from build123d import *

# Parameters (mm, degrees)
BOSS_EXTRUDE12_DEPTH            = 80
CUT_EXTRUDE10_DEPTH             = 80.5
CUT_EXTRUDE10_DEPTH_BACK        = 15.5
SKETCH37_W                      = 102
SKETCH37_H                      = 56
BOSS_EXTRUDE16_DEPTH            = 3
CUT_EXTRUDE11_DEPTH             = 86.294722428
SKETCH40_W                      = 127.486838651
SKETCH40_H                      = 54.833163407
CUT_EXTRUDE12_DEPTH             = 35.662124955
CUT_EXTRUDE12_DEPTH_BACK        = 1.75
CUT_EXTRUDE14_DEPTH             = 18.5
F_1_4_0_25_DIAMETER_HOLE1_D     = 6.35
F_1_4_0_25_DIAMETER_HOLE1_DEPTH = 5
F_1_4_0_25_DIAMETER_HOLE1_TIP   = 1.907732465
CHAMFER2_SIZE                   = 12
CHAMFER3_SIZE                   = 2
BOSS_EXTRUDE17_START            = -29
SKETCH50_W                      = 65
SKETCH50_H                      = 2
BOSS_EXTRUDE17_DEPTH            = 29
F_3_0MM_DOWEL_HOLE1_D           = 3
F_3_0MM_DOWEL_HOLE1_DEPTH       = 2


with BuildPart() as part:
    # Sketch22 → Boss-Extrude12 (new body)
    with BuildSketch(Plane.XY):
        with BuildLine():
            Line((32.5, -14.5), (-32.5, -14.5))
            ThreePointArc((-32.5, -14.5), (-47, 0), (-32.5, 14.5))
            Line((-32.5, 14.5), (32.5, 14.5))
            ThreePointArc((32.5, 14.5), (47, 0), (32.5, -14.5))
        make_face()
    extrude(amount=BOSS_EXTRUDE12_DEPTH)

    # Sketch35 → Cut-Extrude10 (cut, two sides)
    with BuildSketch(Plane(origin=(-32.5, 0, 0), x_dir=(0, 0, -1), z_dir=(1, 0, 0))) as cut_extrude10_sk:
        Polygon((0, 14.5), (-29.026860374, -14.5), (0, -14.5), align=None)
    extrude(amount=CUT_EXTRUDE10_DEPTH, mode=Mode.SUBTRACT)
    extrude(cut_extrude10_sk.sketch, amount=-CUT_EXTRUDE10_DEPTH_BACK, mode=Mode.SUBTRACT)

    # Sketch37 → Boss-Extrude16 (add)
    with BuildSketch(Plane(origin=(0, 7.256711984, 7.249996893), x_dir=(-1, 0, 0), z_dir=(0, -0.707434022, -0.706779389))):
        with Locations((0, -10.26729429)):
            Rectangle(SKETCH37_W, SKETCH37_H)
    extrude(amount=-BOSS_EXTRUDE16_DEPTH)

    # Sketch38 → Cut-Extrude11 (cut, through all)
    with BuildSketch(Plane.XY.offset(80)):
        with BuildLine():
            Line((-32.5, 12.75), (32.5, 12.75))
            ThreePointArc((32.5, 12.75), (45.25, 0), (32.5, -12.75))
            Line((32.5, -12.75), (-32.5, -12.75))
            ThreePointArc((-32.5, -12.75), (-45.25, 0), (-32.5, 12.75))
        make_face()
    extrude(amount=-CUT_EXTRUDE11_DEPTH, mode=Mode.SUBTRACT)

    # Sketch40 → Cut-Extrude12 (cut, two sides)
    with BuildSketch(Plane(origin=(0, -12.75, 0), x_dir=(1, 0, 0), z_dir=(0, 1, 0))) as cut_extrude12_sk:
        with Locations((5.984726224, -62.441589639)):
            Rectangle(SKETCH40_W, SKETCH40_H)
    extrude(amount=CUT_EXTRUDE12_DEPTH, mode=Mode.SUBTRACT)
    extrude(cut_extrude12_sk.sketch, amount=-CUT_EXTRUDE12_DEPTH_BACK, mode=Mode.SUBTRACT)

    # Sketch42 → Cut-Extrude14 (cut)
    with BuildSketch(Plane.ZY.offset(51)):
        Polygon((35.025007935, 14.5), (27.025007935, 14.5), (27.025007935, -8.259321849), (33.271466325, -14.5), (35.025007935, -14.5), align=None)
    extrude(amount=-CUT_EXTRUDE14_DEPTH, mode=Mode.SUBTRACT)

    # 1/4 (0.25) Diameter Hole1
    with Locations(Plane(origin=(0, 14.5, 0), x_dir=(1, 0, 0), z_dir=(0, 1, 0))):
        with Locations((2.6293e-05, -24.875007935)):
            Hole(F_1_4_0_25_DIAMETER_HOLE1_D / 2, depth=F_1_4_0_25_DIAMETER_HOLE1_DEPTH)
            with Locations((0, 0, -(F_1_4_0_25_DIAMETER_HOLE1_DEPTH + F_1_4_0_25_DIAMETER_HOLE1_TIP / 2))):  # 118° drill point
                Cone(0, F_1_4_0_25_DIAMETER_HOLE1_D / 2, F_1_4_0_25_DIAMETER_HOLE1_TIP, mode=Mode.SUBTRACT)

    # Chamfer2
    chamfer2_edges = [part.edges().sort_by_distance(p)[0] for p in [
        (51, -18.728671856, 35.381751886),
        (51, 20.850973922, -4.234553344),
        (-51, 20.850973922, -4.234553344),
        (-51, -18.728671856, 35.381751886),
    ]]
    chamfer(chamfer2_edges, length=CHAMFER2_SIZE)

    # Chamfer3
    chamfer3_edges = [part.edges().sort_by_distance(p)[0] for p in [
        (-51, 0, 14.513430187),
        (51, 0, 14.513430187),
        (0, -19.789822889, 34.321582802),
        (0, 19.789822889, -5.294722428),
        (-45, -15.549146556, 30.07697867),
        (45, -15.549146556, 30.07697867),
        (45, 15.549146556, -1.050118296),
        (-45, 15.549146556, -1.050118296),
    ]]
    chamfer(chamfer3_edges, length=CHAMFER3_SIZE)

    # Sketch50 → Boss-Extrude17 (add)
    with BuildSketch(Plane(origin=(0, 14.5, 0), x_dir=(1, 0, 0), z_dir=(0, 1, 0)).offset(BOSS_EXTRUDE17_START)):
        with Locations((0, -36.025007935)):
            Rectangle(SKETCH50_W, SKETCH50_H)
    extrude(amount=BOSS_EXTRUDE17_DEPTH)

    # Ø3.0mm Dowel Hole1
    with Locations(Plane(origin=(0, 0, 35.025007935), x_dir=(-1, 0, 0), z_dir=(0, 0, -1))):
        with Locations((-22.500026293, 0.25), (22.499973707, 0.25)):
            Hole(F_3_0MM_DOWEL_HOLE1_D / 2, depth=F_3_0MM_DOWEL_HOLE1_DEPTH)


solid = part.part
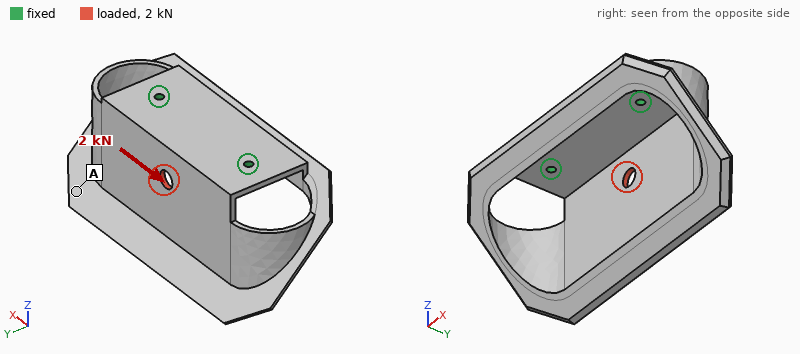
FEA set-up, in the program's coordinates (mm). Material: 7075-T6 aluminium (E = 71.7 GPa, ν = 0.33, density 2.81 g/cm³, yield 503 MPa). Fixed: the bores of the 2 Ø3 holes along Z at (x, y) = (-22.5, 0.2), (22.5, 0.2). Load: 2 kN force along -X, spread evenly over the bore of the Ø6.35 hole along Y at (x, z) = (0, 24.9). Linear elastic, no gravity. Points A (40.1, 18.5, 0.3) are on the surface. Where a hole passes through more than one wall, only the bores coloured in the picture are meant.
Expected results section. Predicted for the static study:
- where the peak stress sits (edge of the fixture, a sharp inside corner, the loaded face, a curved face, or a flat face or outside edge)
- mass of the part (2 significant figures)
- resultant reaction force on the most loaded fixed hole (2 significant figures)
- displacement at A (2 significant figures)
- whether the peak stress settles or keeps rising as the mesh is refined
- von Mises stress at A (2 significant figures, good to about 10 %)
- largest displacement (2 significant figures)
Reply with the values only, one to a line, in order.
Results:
edge of the fixture
44 g
1.3 kN
0.35 mm
keeps rising
27 MPa
0.38 mm
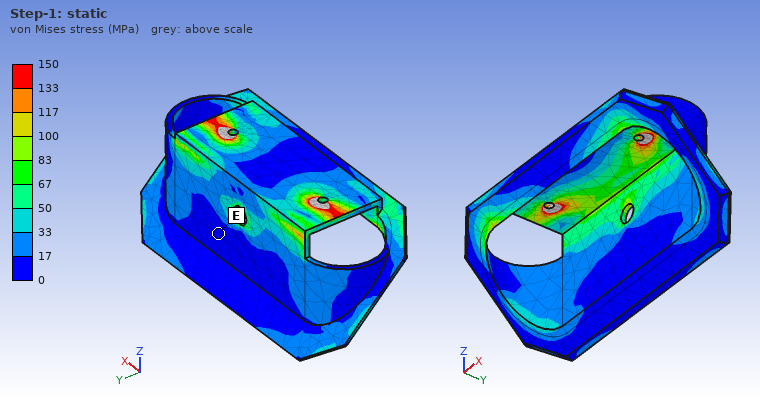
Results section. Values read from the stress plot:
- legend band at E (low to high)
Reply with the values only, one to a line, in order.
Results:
0 to 17 MPa
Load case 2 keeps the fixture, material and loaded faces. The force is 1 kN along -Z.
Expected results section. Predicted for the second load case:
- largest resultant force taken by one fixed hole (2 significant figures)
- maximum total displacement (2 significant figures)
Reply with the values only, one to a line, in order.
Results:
510 N
0.93 mm
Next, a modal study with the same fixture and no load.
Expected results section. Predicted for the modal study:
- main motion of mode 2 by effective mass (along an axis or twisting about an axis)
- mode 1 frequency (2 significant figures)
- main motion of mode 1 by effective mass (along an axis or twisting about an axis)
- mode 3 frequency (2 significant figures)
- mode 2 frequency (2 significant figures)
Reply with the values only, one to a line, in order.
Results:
along X
750 Hz
along Y
2000 Hz
1500 Hz
